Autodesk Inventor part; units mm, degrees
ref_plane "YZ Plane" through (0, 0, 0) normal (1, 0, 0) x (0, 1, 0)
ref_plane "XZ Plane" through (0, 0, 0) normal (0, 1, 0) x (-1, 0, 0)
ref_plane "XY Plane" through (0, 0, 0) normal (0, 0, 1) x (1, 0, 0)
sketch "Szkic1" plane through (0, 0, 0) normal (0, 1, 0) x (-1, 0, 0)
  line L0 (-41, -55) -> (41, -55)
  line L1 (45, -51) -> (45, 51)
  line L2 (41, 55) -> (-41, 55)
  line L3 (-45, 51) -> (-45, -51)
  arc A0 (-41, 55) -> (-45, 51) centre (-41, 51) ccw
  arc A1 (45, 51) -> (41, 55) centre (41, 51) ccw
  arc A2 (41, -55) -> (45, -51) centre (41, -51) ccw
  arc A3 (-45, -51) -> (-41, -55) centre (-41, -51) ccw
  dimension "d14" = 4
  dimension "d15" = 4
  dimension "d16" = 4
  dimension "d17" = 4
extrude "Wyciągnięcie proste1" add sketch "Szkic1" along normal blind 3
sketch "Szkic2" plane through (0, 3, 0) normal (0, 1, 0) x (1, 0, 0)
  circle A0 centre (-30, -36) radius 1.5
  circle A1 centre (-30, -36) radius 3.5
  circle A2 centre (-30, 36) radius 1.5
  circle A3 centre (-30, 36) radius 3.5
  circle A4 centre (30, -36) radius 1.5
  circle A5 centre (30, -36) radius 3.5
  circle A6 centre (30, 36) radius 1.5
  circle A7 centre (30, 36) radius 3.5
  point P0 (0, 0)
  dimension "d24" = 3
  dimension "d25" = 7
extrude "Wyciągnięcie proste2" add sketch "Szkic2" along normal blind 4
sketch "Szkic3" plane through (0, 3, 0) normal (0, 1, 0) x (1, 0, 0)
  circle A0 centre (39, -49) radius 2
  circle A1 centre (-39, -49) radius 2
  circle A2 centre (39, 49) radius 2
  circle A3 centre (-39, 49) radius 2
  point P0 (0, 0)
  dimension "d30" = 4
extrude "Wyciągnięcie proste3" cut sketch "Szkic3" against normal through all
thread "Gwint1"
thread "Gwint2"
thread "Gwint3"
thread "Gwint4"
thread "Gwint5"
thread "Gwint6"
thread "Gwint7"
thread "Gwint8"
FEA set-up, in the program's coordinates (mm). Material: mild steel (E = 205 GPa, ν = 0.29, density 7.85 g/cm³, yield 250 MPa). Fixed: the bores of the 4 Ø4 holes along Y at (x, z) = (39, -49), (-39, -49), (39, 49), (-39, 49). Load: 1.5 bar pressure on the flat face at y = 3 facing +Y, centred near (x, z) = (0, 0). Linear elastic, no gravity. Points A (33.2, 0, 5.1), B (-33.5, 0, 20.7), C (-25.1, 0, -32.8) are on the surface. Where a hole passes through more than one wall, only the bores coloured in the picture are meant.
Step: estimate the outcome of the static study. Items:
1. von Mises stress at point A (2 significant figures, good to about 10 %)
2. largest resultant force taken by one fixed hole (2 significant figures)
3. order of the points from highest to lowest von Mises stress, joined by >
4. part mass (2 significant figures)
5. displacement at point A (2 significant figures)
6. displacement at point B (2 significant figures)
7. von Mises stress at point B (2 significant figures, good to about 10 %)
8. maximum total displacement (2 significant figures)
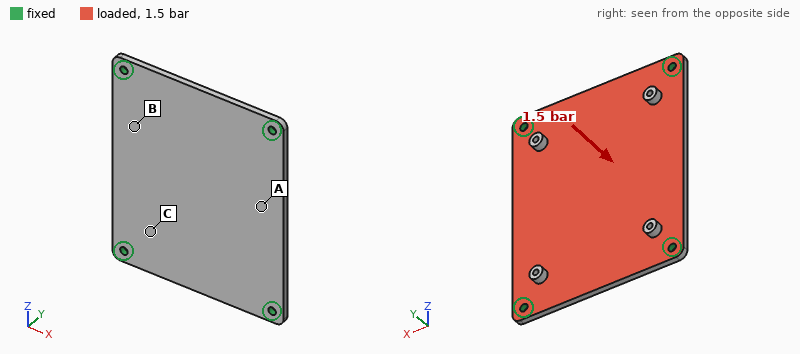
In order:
50 MPa
360 N
A > B > C
240 g
0.12 mm
0.090 mm
31 MPa
0.15 mm
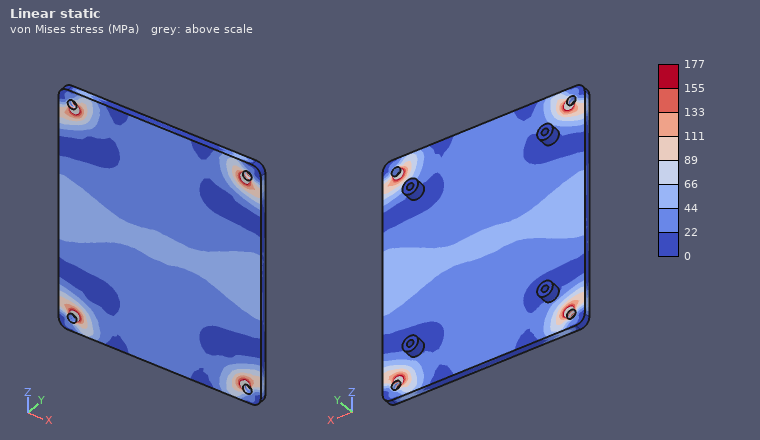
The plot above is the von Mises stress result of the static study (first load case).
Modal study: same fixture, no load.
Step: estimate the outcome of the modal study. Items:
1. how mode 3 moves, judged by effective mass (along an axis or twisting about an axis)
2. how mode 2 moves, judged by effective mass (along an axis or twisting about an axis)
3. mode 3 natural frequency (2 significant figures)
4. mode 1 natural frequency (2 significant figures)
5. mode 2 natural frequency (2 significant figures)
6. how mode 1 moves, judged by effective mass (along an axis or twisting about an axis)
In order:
twisting about X
twisting about Z
2600 Hz
1200 Hz
2000 Hz
along Y
